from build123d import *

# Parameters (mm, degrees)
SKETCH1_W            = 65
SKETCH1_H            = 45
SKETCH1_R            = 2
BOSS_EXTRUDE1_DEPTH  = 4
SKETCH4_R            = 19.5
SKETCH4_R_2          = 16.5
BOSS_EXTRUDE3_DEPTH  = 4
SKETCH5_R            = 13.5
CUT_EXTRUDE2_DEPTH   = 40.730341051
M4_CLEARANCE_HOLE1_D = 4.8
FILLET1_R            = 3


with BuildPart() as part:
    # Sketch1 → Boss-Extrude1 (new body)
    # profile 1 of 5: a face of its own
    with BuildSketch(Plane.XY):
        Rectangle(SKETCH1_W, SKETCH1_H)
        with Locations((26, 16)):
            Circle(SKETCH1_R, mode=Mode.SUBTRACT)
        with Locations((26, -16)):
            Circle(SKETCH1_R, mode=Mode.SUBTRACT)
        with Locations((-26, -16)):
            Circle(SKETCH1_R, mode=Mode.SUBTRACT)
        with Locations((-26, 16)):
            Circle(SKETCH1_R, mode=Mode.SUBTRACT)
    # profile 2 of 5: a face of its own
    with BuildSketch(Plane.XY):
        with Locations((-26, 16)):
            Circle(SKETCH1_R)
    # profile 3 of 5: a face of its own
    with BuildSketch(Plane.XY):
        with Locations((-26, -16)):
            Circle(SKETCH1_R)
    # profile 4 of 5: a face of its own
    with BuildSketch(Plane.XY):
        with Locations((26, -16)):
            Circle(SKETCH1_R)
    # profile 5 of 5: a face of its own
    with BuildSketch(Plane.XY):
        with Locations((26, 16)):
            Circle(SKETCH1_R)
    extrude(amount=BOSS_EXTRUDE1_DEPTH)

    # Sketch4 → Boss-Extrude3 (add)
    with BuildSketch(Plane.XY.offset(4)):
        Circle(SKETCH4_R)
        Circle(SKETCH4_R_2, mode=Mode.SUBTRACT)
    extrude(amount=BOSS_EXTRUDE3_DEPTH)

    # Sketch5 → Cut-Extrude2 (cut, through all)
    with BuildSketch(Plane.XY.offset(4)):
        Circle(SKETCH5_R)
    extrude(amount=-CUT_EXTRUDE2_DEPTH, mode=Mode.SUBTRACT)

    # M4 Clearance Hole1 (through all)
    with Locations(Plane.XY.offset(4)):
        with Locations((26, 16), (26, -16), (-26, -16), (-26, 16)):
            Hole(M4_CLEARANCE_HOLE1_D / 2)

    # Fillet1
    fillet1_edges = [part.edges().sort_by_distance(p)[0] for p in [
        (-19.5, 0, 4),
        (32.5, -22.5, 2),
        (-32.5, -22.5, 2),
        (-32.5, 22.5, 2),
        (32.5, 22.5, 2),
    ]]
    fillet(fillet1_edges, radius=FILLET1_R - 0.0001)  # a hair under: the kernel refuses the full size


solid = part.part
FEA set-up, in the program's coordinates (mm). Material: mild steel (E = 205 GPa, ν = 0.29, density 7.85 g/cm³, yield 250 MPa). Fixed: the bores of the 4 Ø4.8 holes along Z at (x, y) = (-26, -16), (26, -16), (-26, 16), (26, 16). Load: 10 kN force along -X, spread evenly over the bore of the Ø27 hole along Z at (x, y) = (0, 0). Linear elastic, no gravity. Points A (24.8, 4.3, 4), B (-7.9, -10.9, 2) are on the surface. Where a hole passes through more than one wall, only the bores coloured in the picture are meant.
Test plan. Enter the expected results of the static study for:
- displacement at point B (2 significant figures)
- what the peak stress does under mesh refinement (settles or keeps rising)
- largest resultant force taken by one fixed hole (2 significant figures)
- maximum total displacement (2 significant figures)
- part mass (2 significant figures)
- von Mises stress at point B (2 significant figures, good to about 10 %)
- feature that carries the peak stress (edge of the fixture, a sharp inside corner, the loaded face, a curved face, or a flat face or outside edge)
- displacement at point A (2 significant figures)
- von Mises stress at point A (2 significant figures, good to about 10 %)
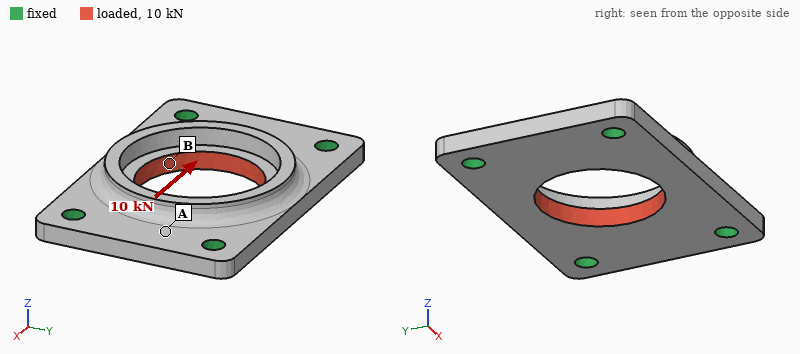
3.6 µm
keeps rising
2.6 kN
4.2 µm
84 g
45 MPa
edge of the fixture
3.0 µm
16 MPa
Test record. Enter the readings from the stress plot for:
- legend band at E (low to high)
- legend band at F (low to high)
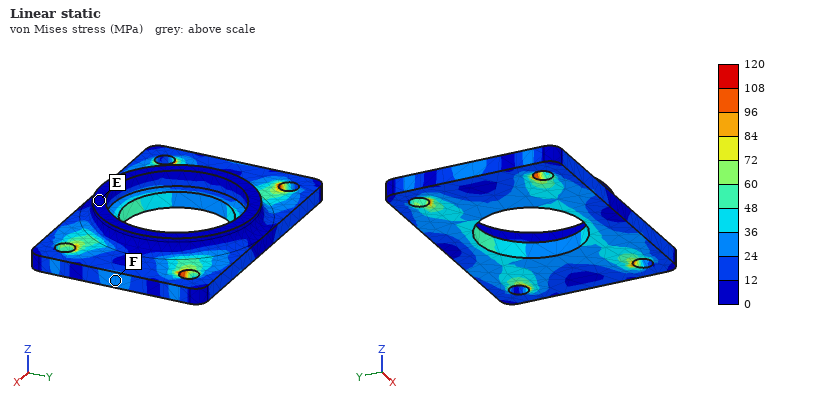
0 to 12 MPa
24 to 36 MPa
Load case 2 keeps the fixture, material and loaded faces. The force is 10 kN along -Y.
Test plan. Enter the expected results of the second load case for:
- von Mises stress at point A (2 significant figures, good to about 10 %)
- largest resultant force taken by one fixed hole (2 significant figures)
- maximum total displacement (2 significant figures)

47 MPa
2.7 kN
13 µm
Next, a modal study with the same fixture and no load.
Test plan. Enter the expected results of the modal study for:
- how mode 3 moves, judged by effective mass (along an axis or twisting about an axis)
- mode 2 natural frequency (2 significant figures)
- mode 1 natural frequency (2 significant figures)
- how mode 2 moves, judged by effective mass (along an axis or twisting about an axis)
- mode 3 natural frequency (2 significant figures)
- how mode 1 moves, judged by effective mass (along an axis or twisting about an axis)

twisting about Y
11 kHz
9500 Hz
twisting about X
18 kHz
along Z
